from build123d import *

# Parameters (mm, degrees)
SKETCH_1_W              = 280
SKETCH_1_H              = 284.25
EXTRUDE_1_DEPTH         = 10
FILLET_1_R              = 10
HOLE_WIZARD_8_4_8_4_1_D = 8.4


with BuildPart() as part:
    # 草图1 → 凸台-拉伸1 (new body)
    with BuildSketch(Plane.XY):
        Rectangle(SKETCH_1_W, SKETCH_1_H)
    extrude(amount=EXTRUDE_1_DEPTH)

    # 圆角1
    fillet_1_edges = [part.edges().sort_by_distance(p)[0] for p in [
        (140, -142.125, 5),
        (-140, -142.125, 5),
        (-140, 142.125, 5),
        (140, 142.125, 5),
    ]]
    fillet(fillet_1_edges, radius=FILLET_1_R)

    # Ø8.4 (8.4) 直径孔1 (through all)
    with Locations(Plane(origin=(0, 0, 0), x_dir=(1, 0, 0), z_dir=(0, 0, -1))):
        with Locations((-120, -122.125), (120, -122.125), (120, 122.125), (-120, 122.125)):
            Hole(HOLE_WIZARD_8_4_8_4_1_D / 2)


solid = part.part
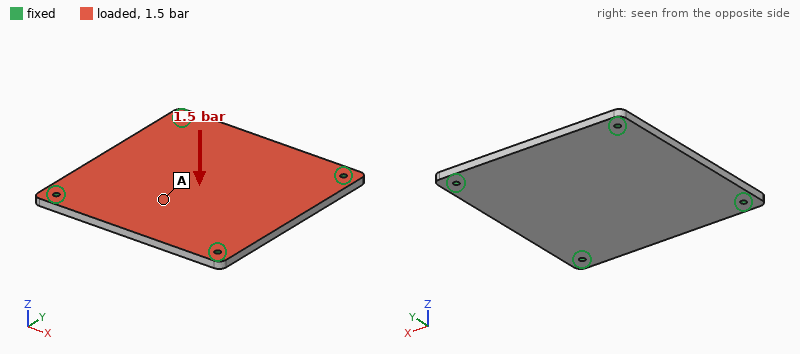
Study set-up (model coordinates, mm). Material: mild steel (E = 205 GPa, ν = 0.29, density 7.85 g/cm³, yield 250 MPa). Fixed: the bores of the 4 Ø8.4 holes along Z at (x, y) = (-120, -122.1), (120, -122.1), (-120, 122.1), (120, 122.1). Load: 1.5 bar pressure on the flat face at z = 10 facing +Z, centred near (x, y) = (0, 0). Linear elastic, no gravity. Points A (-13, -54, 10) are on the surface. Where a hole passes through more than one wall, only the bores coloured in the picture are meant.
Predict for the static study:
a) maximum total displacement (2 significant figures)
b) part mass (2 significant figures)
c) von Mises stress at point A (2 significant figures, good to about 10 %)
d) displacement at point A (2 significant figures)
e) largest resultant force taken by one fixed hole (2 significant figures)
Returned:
0.24 mm
6.2 kg
28 MPa
0.21 mm
3.0 kN
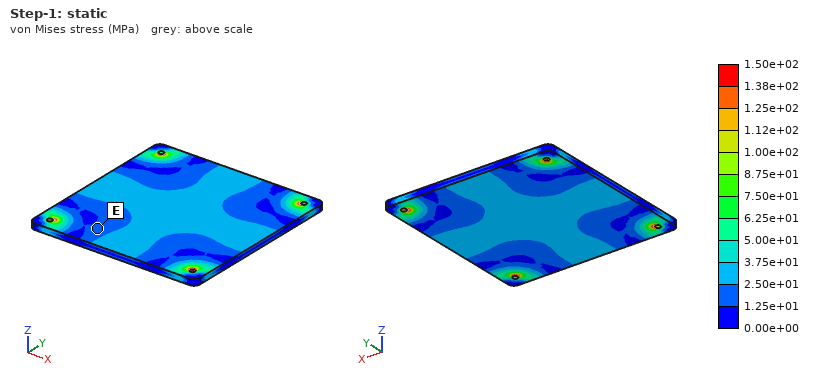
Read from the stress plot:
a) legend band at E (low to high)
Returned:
1.25e+01 to 2.50e+01 MPa
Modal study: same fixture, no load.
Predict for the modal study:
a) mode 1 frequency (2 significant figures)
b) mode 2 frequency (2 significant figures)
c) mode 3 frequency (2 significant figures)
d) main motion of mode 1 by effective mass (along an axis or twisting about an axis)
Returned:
540 Hz
930 Hz
950 Hz
along Z
